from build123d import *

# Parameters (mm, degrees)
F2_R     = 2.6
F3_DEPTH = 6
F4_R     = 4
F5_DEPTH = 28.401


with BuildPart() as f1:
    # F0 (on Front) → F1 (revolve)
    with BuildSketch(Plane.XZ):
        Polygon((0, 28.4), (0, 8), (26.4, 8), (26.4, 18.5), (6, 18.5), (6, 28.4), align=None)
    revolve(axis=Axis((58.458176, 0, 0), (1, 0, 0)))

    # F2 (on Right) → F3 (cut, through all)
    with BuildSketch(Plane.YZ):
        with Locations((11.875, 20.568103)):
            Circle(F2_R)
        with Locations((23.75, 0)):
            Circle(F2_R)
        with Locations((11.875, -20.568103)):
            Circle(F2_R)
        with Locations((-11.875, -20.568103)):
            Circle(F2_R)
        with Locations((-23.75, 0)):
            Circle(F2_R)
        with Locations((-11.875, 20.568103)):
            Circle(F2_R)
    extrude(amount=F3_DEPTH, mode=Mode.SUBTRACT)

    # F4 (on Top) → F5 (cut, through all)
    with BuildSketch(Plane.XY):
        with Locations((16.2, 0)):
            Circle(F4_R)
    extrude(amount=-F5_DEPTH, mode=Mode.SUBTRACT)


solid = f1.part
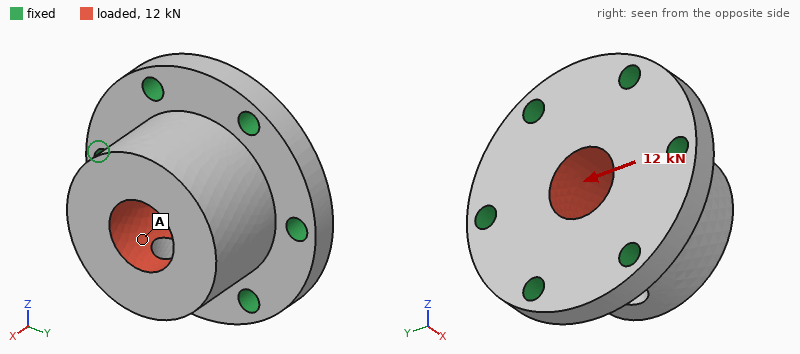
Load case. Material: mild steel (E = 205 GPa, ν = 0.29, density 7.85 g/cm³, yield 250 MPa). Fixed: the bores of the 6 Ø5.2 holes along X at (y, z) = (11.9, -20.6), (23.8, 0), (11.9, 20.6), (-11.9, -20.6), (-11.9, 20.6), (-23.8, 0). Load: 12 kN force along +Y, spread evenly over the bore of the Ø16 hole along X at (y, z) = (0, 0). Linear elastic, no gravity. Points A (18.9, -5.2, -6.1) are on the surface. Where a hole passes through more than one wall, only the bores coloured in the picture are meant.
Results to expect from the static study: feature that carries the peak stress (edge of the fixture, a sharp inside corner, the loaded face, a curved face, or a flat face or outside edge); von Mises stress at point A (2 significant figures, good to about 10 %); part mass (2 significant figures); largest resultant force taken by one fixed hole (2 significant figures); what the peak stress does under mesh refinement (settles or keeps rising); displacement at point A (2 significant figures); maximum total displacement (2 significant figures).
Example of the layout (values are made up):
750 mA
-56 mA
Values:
edge of the fixture
18 MPa
240 g
3.4 kN
keeps rising
5.6 µm
7.8 µm
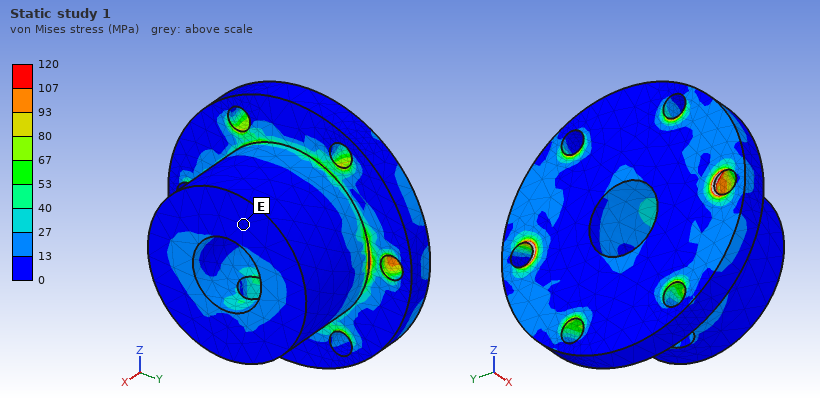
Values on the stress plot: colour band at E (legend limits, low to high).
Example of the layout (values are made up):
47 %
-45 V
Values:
0 to 13 MPa
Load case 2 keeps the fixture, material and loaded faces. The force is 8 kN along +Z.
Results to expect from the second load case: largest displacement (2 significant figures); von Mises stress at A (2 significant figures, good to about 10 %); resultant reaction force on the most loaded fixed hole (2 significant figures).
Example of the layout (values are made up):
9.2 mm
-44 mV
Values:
5.0 µm
13 MPa
2.0 kN
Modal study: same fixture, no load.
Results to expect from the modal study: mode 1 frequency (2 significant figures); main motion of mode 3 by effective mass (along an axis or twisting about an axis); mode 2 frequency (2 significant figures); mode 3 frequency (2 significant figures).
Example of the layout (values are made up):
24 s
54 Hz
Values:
17 kHz
along X
18 kHz
21 kHz
